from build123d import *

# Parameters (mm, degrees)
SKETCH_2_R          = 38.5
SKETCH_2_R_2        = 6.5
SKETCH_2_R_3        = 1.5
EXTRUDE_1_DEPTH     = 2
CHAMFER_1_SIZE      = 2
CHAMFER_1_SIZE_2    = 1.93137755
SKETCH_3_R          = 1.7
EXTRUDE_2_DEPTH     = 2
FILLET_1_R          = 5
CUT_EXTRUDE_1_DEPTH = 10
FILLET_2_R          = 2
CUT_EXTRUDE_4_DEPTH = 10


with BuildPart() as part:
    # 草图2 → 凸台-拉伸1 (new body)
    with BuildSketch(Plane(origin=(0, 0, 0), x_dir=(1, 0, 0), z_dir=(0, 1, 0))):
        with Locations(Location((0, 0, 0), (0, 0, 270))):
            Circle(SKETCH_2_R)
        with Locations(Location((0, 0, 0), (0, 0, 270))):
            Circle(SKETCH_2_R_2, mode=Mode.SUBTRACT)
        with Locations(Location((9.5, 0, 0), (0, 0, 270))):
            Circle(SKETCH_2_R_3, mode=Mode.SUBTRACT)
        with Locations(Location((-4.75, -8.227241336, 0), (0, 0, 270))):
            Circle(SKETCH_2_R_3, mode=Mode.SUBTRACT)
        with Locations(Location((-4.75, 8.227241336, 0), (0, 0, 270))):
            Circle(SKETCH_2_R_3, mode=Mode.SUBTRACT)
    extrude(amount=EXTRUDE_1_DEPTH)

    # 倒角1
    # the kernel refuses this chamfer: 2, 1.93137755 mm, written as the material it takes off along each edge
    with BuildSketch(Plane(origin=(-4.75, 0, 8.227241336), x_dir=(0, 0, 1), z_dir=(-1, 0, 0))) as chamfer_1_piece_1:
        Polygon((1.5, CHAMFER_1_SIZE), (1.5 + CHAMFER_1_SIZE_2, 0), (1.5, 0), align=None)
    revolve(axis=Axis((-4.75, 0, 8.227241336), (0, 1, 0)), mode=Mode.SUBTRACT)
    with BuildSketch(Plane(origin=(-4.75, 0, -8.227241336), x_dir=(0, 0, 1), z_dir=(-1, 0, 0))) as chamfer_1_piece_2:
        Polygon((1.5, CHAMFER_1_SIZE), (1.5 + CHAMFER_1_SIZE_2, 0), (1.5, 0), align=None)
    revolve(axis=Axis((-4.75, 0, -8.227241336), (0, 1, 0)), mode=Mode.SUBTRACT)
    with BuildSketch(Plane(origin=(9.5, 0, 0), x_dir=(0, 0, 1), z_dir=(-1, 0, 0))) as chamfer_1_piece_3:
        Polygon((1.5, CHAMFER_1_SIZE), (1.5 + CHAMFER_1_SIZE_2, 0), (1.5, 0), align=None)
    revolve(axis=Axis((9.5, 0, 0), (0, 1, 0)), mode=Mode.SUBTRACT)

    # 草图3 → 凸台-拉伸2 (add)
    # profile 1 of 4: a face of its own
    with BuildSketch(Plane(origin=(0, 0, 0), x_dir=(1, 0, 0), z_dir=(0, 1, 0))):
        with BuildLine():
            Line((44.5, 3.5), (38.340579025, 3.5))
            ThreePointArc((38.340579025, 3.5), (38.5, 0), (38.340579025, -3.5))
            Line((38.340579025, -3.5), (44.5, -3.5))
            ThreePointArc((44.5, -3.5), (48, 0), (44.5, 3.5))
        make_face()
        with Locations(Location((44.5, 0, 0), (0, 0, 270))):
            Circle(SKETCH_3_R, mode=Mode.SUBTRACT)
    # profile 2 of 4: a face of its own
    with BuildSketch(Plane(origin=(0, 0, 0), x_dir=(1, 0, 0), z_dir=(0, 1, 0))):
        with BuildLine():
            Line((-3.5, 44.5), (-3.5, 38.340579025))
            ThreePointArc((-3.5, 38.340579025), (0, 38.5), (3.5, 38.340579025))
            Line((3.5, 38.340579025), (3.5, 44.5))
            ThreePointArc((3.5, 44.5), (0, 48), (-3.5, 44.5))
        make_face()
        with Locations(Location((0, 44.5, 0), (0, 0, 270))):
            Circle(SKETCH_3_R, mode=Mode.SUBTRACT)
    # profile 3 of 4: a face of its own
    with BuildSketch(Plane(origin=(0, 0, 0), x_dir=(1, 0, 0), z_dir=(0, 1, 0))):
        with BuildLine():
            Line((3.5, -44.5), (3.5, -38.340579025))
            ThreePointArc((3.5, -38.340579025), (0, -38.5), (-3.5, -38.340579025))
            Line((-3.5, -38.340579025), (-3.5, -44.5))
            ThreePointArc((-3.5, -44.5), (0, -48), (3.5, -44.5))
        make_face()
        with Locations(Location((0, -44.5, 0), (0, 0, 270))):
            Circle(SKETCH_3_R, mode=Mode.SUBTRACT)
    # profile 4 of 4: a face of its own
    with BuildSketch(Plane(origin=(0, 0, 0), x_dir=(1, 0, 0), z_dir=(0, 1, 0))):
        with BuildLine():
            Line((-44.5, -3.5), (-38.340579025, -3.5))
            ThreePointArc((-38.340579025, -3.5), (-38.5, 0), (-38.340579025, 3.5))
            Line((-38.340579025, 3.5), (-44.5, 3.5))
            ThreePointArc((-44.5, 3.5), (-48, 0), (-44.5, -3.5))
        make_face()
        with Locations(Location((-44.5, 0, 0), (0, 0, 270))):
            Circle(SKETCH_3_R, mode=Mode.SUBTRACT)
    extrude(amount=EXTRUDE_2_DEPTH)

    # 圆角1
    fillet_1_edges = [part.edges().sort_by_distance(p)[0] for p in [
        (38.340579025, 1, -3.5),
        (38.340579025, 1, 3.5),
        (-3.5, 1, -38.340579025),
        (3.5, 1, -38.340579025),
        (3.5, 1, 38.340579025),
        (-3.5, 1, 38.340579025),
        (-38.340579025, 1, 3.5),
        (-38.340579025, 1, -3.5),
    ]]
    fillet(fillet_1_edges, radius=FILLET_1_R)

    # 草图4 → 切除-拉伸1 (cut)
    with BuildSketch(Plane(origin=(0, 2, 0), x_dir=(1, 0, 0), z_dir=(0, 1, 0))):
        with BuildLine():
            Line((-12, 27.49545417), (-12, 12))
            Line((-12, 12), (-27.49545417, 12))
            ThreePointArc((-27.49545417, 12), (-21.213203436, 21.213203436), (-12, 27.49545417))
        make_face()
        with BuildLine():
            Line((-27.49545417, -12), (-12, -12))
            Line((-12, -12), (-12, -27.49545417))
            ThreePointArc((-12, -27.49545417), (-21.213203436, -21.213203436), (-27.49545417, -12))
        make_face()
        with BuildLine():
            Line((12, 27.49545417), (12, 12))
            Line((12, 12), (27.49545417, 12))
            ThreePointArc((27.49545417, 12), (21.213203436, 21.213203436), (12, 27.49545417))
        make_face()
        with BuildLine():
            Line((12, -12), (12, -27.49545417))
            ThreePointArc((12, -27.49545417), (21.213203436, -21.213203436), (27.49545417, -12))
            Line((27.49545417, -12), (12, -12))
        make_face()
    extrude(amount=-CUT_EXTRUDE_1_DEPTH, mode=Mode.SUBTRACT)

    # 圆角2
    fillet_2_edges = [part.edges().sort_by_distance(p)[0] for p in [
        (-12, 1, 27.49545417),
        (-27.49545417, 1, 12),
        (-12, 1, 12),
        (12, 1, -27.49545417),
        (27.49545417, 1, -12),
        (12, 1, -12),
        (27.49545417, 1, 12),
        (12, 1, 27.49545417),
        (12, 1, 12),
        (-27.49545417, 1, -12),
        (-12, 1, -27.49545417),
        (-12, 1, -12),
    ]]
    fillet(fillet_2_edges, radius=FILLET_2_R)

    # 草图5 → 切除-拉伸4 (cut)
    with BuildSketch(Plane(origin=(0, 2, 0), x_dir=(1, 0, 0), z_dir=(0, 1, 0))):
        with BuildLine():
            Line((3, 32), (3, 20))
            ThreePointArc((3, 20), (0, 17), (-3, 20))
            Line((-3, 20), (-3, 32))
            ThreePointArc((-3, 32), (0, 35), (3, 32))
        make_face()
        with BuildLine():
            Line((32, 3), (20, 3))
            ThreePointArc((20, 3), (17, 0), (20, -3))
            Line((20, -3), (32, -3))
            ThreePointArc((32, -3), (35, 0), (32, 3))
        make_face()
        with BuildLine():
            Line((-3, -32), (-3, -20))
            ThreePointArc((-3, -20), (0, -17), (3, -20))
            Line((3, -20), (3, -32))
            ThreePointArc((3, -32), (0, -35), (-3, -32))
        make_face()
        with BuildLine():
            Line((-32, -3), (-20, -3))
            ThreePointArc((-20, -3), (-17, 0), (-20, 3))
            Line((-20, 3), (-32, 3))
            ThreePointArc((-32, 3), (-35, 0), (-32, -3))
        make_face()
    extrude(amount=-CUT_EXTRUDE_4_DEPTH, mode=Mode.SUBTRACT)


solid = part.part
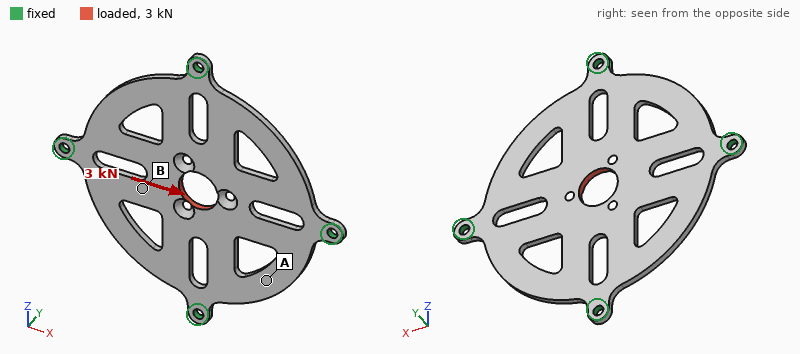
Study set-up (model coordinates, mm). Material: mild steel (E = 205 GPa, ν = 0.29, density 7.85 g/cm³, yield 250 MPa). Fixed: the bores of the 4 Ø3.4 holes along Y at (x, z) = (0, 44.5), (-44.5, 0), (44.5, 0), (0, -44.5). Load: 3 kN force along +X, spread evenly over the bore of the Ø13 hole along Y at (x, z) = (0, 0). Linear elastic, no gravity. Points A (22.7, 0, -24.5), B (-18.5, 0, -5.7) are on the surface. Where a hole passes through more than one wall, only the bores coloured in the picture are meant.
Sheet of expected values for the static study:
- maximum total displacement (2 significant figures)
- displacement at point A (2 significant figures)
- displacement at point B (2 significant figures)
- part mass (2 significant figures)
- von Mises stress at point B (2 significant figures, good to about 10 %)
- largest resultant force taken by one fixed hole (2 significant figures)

17 µm
6.6 µm
8.4 µm
58 g
39 MPa
1.2 kN
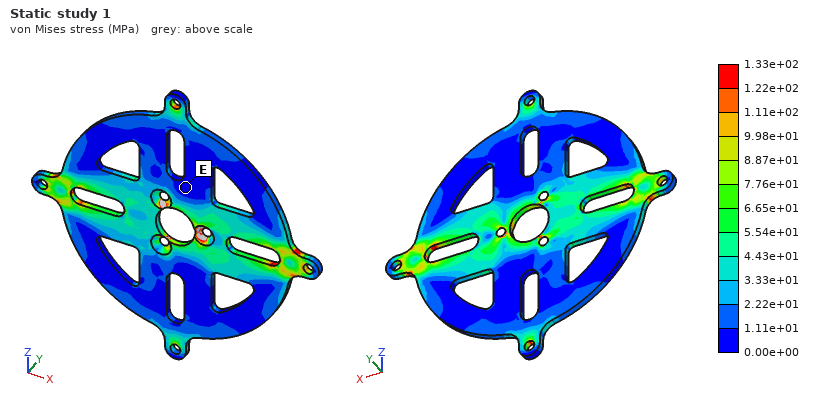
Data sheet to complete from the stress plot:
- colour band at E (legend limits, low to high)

0.00e+00 to 1.11e+01 MPa
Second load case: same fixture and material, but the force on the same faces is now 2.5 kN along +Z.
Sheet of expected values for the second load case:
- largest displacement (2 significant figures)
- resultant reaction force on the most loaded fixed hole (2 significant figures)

14 µm
970 N
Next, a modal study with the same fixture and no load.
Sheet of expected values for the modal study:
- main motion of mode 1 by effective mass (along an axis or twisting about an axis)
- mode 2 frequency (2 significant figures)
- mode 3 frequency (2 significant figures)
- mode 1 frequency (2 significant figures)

along Y
2500 Hz
2500 Hz
1500 Hz
